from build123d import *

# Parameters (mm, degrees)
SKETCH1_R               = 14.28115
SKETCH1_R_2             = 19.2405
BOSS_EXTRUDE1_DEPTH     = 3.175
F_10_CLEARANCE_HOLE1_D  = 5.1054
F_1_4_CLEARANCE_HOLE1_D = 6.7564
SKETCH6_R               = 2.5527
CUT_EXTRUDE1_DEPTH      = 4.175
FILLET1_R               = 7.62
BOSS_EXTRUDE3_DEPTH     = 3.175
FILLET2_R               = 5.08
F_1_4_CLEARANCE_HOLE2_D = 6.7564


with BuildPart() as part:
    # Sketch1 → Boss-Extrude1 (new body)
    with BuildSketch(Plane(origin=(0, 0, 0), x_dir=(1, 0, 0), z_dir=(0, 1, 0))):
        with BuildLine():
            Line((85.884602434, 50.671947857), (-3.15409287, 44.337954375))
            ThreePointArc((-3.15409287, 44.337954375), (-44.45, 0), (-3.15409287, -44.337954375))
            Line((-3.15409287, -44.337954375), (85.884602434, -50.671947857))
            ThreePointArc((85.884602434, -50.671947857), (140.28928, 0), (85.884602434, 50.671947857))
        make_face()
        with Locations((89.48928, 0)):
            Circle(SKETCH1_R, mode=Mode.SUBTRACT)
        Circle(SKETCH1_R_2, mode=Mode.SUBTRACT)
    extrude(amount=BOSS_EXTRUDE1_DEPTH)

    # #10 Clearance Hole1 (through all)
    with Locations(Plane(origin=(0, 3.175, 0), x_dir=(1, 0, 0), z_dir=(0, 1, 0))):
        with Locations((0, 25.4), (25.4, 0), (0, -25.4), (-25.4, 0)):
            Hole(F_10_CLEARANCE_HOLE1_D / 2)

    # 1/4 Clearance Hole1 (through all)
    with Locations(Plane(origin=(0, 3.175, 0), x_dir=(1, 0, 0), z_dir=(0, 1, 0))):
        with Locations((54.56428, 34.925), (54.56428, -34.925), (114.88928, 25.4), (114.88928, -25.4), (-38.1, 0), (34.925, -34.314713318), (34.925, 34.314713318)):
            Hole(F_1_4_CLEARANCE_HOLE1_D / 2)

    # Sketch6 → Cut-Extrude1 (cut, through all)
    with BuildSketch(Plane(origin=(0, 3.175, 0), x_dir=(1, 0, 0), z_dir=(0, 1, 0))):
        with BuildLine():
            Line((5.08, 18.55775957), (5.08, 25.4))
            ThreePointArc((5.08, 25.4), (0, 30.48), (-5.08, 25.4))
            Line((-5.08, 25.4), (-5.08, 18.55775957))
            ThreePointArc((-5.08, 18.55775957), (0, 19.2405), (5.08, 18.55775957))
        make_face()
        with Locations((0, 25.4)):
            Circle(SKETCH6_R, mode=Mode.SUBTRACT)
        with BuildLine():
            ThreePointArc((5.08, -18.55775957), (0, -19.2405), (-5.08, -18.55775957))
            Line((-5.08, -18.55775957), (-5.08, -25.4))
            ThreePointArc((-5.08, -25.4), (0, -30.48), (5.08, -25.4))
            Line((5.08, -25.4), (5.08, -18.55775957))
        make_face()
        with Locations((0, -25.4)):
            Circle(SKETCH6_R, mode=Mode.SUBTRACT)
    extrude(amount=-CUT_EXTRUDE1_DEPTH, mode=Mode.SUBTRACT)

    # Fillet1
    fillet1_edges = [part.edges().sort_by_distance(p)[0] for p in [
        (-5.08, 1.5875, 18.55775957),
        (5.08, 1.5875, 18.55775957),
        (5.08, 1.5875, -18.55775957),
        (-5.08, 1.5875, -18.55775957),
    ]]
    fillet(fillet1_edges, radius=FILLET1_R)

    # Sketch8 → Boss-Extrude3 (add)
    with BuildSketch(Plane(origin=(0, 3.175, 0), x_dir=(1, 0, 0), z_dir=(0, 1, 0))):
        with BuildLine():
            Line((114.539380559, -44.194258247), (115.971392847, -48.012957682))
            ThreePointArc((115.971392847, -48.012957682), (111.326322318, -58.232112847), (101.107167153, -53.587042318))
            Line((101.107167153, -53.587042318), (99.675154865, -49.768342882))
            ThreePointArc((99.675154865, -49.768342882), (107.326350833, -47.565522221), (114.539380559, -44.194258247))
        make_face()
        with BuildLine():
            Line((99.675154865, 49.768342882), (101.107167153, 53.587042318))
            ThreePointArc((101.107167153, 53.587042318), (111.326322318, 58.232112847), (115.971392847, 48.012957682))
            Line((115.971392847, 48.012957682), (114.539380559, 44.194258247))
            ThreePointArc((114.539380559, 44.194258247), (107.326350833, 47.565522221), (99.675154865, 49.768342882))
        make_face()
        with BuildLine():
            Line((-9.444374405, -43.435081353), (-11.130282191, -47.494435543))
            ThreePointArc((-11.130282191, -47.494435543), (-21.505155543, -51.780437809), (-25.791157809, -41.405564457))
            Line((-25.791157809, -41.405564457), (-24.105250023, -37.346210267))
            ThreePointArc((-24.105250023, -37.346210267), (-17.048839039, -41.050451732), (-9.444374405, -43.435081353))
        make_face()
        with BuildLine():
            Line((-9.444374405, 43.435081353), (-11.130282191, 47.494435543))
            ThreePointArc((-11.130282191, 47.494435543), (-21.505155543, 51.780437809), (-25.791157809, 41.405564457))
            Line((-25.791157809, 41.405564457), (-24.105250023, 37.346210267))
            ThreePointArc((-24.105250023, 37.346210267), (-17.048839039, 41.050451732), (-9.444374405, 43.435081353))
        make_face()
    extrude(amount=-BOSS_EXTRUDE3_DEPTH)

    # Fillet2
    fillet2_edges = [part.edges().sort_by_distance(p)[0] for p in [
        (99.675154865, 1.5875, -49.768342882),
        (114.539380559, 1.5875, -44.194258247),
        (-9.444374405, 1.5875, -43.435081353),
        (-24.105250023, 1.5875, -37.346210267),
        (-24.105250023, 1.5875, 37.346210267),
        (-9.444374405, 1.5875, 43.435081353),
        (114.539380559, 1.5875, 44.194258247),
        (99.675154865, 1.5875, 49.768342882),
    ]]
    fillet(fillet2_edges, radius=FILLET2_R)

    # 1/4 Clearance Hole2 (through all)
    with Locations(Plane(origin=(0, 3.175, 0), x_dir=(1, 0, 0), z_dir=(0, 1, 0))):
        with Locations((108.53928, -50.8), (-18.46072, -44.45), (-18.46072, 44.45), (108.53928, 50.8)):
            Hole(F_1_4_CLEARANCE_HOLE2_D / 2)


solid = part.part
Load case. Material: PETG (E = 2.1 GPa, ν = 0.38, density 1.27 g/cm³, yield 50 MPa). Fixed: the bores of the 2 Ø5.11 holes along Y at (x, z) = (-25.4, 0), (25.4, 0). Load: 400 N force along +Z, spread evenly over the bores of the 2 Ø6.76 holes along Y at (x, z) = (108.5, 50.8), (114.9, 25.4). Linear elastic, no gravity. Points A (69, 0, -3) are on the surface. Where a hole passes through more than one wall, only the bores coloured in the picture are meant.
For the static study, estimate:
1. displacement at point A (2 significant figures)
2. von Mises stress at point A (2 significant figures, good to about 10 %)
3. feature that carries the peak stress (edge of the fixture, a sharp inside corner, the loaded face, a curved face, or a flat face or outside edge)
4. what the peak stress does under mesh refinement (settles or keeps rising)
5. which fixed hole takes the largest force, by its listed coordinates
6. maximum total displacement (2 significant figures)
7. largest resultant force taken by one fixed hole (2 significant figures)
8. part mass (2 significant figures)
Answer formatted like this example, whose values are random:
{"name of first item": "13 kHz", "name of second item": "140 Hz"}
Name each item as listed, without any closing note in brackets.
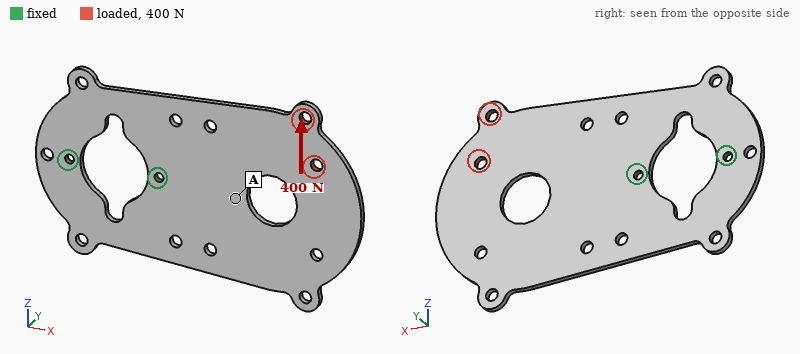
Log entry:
{"displacement at point A": "0.84 mm", "von Mises stress at point A": "4.7 MPa", "feature that carries the peak stress": "edge of the fixture", "what the peak stress does under mesh refinement": "keeps rising", "which fixed hole takes the largest force, by its listed coordinates": "(25.4, 0)", "maximum total displacement": "2.3 mm", "largest resultant force taken by one fixed hole": "960 N", "part mass": "56 g"}
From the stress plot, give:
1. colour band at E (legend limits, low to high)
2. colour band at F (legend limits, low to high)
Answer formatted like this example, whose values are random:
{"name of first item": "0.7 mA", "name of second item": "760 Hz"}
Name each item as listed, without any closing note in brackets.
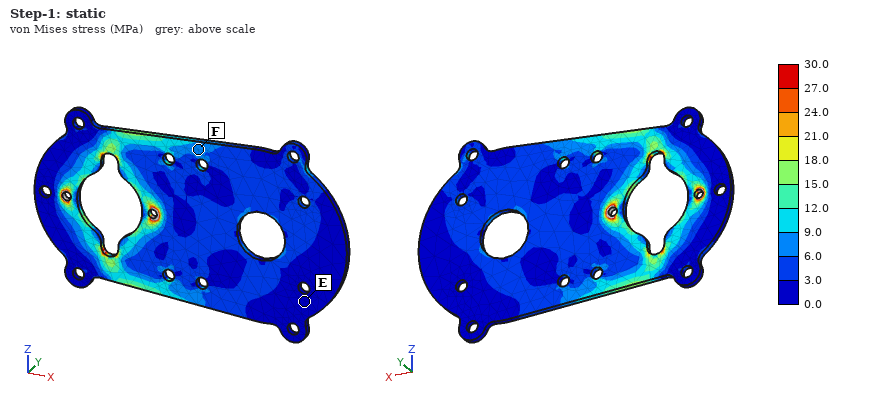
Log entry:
{"colour band at E": "0.0 to 3.0 MPa", "colour band at F": "6.0 to 9.0 MPa"}
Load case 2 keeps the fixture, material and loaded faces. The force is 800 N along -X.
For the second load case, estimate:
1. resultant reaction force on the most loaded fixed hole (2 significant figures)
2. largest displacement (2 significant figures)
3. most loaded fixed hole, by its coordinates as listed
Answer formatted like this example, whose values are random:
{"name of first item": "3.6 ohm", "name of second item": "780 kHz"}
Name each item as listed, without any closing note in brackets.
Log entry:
{"resultant reaction force on the most loaded fixed hole": "820 N", "largest displacement": "2.0 mm", "most loaded fixed hole, by its coordinates as listed": "(25.4, 0)"}
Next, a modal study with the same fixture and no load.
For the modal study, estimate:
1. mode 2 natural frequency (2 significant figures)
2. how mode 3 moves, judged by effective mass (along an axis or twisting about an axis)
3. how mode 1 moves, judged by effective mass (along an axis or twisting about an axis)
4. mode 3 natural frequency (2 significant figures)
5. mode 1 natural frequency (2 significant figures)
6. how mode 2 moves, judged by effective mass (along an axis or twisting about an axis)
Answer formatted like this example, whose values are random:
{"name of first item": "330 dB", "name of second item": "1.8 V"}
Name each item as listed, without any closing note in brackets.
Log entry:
{"mode 2 natural frequency": "99 Hz", "how mode 3 moves, judged by effective mass": "along Y", "how mode 1 moves, judged by effective mass": "along Y", "mode 3 natural frequency": "240 Hz", "mode 1 natural frequency": "51 Hz", "how mode 2 moves, judged by effective mass": "twisting about X"}
